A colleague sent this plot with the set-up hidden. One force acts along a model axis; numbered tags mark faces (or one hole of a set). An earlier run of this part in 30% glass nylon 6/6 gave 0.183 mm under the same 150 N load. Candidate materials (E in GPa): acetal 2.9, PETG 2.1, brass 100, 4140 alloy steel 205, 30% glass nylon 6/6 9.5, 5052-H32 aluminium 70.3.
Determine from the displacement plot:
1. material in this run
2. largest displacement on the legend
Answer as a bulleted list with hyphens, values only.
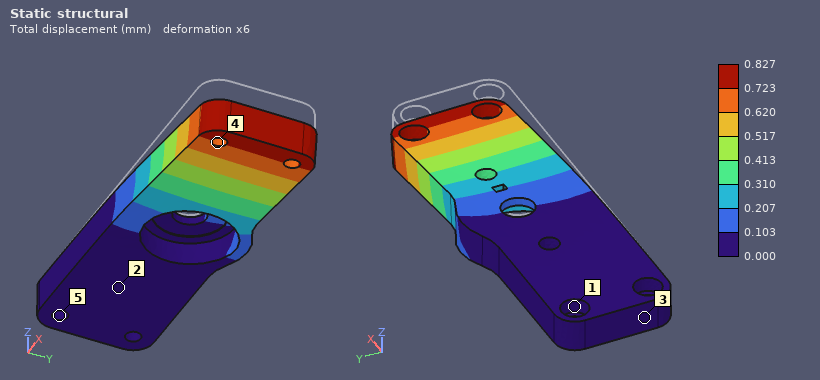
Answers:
- PETG
- 0.827 mm
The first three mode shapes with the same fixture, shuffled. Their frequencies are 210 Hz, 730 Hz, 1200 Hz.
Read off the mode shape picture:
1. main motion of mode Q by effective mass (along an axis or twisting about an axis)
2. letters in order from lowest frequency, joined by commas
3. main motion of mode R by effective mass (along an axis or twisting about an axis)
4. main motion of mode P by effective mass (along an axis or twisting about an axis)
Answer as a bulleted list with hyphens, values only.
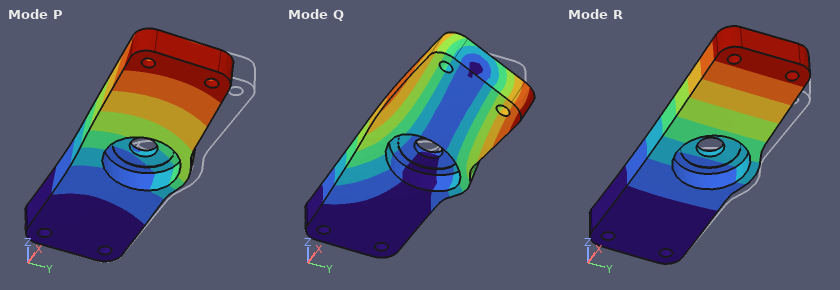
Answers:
- twisting about X
- R, P, Q
- along Z
- along Y
